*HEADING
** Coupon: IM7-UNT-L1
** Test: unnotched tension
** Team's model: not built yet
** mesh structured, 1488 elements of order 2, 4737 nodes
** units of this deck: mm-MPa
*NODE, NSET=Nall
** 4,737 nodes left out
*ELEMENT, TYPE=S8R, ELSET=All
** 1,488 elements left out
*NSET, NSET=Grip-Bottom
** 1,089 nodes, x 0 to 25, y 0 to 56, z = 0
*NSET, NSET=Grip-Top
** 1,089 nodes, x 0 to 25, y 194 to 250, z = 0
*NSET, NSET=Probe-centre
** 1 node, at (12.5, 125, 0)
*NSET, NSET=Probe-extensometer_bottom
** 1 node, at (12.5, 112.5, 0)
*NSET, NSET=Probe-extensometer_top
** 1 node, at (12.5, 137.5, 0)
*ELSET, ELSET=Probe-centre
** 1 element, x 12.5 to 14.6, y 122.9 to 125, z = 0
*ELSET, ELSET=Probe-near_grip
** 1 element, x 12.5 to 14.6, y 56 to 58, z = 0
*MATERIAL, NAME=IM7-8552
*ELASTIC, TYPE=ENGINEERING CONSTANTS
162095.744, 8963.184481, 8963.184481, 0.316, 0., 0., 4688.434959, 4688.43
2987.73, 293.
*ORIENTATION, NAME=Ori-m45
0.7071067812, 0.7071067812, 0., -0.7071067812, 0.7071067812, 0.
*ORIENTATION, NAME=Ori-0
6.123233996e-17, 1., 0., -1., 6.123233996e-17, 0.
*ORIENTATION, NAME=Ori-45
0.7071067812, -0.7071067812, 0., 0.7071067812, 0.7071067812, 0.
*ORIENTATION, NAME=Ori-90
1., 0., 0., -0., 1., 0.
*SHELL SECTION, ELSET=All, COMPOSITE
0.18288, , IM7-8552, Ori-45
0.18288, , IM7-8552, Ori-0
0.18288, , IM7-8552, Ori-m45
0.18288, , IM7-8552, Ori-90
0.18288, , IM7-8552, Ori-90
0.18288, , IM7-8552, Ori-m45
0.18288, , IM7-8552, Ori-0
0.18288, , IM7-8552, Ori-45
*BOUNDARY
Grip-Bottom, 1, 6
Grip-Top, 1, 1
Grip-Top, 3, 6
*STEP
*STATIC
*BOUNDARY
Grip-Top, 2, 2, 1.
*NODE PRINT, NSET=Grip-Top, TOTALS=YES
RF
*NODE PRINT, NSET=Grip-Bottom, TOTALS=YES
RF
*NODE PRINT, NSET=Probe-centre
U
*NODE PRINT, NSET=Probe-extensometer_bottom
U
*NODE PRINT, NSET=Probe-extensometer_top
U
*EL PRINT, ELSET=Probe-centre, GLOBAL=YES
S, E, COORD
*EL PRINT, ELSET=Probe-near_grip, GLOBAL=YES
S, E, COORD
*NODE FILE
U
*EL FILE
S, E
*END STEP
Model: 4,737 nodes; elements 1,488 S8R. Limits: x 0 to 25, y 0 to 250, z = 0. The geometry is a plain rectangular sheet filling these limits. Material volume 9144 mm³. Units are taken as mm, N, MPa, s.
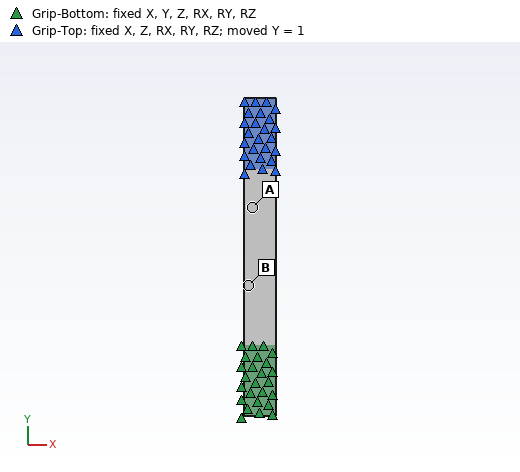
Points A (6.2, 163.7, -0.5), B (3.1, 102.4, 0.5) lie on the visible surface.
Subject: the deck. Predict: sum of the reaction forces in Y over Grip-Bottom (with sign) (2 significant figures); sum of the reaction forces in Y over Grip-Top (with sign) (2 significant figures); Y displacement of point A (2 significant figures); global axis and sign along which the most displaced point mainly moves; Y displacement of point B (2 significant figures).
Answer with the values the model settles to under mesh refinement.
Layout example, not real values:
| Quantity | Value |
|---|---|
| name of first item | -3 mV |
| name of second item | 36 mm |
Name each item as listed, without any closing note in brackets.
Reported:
| Quantity | Value |
|---|---|
| sum of the reaction forces in Y over Grip-Bottom (with sign) | -16000 N |
| sum of the reaction forces in Y over Grip-Top (with sign) | 16000 N |
| Y displacement of point A | 0.78 mm |
| global axis and sign along which the most displaced point mainly moves | +Y |
| Y displacement of point B | 0.34 mm |
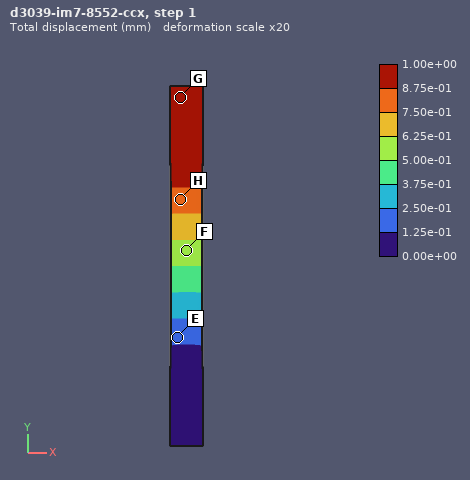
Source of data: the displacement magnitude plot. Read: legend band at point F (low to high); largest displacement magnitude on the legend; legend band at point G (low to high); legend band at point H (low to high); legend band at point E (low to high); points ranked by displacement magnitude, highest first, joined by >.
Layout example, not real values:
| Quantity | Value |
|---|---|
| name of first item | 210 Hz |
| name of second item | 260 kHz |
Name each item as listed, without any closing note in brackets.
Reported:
| Quantity | Value |
|---|---|
| legend band at point F | 5.00e-01 to 6.25e-01 mm |
| largest displacement magnitude on the legend | 1.00e+00 mm |
| legend band at point G | 8.75e-01 to 1.00e+00 mm |
| legend band at point H | 7.50e-01 to 8.75e-01 mm |
| legend band at point E | 1.25e-01 to 2.50e-01 mm |
| points ranked by displacement magnitude, highest first, joined by > | G > H > F > E |
